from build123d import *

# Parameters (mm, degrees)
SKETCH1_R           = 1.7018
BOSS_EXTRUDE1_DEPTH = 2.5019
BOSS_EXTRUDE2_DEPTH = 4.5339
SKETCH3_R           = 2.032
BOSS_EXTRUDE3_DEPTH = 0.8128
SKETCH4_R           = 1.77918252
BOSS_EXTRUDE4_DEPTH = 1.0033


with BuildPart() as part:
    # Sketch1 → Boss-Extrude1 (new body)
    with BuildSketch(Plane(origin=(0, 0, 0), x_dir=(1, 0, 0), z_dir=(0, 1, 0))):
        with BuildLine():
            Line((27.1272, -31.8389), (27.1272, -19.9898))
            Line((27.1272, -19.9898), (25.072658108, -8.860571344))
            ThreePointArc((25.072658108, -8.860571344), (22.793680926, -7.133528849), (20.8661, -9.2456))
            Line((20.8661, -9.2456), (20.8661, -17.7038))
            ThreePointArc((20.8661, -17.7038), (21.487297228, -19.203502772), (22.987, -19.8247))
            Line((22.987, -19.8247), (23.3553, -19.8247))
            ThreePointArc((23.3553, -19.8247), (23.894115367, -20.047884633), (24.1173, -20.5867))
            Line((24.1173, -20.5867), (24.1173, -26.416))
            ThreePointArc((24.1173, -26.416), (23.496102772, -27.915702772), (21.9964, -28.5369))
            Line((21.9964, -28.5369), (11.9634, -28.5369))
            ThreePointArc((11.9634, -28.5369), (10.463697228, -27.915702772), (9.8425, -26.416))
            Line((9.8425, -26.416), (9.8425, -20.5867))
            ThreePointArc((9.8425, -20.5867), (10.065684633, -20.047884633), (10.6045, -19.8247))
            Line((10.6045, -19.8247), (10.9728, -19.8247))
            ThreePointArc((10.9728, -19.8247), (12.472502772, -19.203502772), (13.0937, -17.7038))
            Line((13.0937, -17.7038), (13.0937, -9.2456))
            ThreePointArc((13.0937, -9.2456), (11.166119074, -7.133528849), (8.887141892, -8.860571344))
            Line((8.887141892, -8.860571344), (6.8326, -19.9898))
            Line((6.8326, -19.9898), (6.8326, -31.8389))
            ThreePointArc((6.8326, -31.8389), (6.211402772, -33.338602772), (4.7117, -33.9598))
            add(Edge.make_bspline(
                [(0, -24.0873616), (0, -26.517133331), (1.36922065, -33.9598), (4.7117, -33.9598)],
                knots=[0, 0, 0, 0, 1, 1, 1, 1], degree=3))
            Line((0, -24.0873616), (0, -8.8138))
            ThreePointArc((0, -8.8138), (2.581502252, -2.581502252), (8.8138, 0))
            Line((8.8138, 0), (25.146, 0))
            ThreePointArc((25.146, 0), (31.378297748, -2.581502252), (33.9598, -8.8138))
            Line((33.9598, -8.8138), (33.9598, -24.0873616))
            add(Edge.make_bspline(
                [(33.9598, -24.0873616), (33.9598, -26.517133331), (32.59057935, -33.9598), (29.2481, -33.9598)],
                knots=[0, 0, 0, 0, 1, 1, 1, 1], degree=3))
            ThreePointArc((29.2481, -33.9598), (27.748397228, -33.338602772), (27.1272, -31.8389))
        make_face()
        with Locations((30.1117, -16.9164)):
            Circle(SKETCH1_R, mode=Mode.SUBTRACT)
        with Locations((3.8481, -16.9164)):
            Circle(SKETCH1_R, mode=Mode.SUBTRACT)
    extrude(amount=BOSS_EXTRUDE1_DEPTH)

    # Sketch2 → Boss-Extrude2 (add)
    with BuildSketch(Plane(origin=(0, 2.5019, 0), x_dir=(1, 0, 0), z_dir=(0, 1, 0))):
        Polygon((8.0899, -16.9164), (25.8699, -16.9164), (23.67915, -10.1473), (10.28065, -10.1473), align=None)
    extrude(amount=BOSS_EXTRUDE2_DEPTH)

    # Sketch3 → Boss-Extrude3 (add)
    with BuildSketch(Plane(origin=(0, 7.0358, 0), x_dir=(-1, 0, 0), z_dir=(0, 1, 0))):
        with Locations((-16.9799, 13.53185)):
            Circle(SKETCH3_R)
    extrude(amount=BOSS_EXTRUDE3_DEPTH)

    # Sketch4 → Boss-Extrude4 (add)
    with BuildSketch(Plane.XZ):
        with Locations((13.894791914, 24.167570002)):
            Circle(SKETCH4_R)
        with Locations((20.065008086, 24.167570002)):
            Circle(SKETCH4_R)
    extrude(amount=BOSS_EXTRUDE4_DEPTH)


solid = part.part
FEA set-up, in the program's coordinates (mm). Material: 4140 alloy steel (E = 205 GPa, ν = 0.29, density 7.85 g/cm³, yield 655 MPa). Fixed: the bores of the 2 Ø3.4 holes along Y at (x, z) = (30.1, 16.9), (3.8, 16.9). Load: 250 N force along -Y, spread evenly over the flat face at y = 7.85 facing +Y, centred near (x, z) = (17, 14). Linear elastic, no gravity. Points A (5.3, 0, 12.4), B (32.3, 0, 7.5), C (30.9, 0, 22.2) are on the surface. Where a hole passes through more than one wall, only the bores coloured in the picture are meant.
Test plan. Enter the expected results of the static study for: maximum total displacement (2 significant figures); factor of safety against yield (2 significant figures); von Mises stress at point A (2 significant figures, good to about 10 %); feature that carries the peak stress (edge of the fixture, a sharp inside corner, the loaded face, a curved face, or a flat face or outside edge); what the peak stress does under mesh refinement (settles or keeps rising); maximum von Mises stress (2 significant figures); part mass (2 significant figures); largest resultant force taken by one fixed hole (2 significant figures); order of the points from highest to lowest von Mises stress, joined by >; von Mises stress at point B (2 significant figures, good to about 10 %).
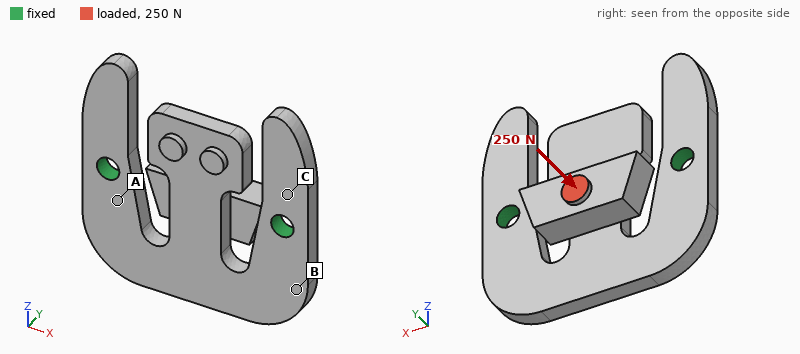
0.20 mm
2.0
75 MPa
a curved face
settles
320 MPa
20 g
130 N
A > B > C
44 MPa
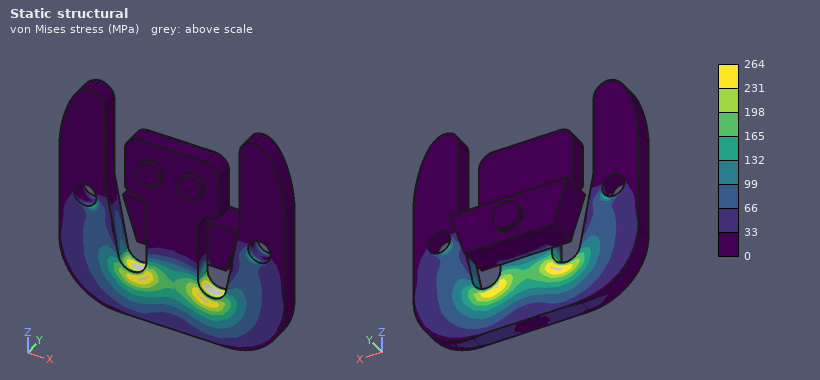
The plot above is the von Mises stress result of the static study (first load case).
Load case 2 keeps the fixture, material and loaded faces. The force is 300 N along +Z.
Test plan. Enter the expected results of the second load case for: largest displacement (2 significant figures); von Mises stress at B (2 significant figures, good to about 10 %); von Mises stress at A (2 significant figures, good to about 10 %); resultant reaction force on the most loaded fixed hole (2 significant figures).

0.26 mm
85 MPa
110 MPa
170 N
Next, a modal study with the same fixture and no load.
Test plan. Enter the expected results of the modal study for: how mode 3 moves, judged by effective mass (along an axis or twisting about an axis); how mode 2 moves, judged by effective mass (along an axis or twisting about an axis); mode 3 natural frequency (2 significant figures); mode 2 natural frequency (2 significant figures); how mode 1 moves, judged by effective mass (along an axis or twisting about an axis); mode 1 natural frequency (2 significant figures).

along X
along Y
6300 Hz
5200 Hz
along Y
1900 Hz
